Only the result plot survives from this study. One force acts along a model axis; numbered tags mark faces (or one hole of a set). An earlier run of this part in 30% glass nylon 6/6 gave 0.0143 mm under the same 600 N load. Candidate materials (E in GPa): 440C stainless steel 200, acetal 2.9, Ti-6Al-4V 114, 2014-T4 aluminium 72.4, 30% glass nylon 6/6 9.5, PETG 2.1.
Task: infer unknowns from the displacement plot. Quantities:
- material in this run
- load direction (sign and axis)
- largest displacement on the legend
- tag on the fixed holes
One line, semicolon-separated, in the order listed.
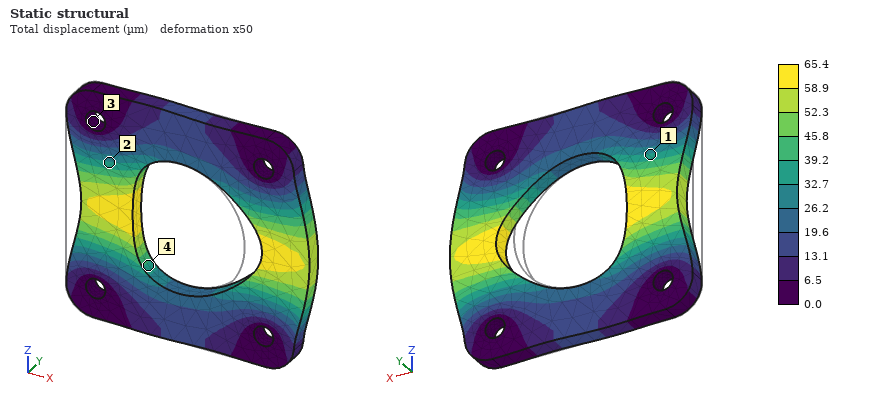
PETG; +X; 65.4 µm; 3
